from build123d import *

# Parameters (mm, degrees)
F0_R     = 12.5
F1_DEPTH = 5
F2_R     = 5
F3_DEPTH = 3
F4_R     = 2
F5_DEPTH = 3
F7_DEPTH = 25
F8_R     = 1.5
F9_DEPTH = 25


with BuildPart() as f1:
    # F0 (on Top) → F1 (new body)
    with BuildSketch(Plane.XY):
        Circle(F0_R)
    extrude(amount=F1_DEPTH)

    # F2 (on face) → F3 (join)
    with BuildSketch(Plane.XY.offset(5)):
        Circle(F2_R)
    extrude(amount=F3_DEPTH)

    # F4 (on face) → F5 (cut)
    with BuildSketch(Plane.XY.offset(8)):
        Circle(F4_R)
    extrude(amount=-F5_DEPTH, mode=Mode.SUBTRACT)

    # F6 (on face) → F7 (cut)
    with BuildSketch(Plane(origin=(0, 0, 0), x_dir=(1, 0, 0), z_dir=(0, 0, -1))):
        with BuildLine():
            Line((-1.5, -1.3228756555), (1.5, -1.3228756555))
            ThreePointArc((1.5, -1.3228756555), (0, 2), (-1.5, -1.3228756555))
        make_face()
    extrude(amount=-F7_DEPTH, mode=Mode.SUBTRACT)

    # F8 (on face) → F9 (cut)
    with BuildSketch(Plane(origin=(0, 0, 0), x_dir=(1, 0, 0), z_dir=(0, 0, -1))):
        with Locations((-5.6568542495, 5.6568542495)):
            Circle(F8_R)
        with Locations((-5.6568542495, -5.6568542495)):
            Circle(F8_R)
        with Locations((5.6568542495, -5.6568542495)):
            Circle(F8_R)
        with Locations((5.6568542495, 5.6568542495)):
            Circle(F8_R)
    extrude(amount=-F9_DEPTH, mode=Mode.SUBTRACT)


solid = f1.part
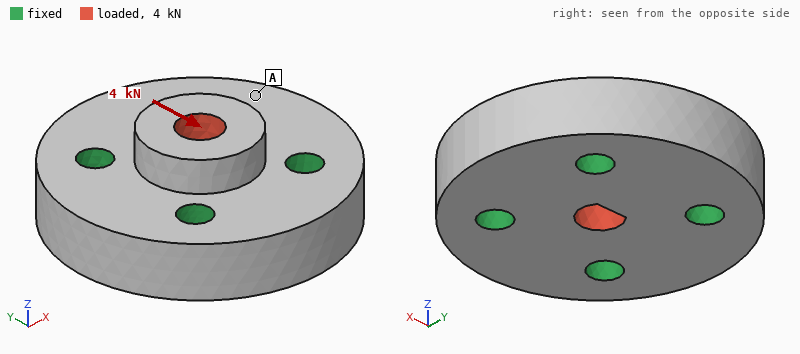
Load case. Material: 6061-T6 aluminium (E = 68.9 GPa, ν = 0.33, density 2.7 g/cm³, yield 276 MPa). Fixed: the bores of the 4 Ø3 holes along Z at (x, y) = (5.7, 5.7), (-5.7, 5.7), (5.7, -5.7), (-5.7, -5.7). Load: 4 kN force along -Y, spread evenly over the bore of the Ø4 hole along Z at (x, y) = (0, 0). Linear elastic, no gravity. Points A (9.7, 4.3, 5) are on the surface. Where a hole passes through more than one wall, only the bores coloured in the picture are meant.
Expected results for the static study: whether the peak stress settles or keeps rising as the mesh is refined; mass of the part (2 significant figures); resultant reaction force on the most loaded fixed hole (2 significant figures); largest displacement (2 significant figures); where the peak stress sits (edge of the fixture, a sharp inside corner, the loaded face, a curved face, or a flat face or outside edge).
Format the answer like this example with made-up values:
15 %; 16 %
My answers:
keeps rising; 6.6 g; 1.2 kN; 9.3 µm; edge of the fixture
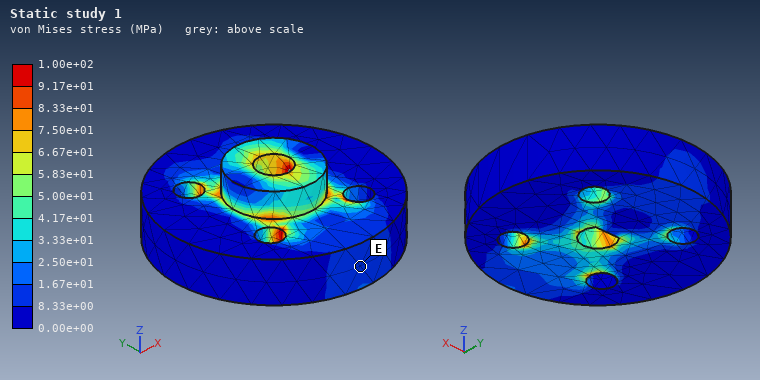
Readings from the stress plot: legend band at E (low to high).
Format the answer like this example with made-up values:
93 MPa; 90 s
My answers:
8.33e+00 to 1.67e+01 MPa
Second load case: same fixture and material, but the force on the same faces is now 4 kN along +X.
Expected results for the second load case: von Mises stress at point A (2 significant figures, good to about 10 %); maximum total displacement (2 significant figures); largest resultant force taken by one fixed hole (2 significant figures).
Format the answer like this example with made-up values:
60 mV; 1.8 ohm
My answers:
12 MPa; 9.1 µm; 1.2 kN
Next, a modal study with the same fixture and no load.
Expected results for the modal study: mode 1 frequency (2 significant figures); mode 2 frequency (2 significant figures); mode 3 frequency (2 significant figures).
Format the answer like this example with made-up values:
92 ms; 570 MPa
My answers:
76 kHz; 78 kHz; 78 kHz
